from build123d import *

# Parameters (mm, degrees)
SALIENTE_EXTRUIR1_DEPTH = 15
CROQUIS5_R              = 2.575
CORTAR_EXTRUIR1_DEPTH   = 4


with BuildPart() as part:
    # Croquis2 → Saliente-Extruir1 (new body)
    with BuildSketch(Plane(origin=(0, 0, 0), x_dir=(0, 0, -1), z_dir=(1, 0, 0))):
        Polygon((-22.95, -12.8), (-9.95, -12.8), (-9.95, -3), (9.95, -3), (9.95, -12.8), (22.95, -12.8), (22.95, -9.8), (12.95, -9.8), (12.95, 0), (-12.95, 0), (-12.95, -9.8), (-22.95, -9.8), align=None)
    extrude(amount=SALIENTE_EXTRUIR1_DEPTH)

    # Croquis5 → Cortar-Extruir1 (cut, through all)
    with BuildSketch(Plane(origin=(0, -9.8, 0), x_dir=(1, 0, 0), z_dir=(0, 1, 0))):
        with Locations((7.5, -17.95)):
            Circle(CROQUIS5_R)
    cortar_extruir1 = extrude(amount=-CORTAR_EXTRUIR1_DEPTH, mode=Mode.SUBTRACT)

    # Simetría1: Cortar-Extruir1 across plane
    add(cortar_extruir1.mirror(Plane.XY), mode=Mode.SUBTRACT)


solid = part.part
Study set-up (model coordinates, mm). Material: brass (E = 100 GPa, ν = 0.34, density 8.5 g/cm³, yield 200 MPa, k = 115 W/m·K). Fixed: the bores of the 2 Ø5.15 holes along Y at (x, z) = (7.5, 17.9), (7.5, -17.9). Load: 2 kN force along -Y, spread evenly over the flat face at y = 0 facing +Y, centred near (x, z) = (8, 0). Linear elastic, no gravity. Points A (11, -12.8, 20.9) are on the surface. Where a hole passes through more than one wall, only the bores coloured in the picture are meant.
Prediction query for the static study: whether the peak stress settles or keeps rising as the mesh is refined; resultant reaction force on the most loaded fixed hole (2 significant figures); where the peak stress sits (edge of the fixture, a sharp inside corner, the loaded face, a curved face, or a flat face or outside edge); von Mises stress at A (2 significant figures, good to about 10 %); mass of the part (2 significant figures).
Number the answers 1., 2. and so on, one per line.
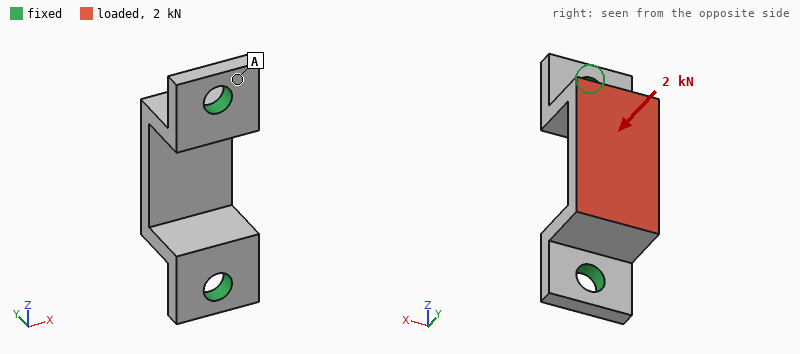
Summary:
1. keeps rising
2. 1.1 kN
3. edge of the fixture
4. 20 MPa
5. 24 g
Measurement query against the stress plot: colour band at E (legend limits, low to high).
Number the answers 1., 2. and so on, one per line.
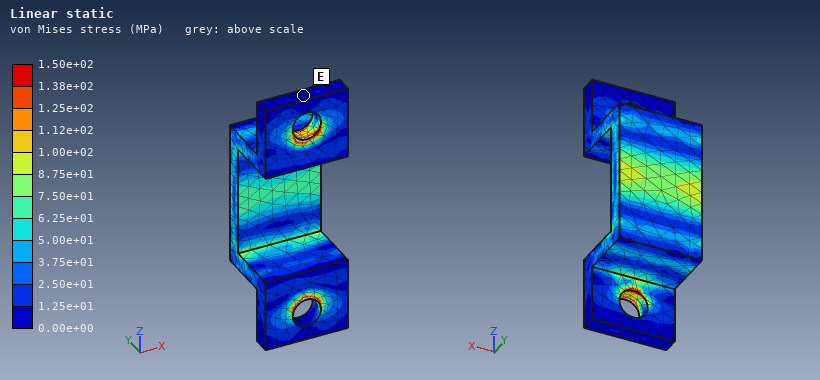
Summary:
1. 0.00e+00 to 1.25e+01 MPa
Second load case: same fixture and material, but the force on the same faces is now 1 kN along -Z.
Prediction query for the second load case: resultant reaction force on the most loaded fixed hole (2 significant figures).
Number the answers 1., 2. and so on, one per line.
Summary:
1. 570 N
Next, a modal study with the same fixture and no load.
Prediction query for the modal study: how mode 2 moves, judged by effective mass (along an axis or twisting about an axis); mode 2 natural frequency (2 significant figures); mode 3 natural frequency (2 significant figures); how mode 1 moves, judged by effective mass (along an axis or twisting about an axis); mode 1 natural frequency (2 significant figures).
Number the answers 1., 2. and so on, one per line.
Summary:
1. along Z
2. 8300 Hz
3. 11 kHz
4. along X
5. 6800 Hz
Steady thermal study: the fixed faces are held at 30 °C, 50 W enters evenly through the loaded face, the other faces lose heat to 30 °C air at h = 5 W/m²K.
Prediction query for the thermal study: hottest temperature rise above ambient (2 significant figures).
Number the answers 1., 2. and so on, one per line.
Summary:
1. 87 K
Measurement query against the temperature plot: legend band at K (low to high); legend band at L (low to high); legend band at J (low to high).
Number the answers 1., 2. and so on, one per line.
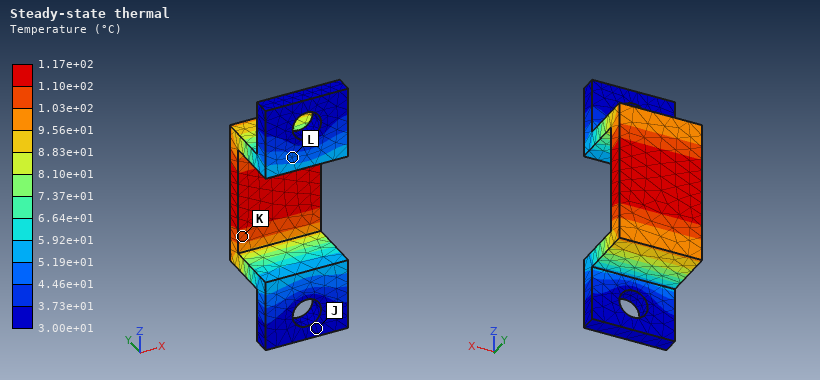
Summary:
1. 1.03e+02 to 1.10e+02 °C
2. 4.46e+01 to 5.19e+01 °C
3. 3.00e+01 to 3.73e+01 °C
